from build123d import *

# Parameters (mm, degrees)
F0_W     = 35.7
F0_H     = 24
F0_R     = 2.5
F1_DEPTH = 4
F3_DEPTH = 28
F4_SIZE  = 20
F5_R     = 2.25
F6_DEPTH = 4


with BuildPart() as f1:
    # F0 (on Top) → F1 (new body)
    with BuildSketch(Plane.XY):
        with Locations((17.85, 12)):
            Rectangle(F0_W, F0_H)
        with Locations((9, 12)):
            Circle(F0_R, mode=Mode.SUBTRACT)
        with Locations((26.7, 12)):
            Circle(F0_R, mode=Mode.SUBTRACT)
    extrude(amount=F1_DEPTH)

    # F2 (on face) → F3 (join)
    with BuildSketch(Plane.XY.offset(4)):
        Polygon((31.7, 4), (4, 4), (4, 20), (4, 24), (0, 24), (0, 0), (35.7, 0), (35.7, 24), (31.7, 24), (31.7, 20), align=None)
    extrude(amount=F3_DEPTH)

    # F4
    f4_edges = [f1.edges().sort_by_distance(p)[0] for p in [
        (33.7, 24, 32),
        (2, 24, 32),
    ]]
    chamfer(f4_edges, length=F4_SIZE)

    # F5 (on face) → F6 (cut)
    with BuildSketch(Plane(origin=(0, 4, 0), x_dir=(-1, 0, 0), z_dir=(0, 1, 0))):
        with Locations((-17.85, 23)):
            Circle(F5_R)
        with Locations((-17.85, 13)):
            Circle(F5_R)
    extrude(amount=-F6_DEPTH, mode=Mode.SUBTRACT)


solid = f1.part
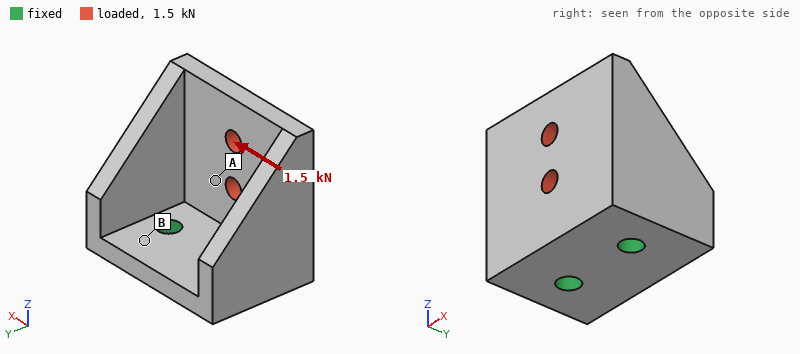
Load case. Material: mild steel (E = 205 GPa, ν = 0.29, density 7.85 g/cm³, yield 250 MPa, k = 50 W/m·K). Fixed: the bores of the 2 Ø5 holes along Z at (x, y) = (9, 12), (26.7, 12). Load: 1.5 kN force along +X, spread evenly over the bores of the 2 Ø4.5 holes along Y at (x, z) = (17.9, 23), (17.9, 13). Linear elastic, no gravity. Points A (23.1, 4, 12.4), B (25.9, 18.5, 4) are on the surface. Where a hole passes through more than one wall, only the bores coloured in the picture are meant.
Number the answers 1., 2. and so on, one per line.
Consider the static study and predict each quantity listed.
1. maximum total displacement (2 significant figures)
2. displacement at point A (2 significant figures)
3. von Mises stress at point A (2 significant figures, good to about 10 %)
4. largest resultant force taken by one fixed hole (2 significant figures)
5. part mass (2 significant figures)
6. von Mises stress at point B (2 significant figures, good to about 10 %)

1. 27 µm
2. 9.4 µm
3. 42 MPa
4. 1.4 kN
5. 79 g
6. 18 MPa
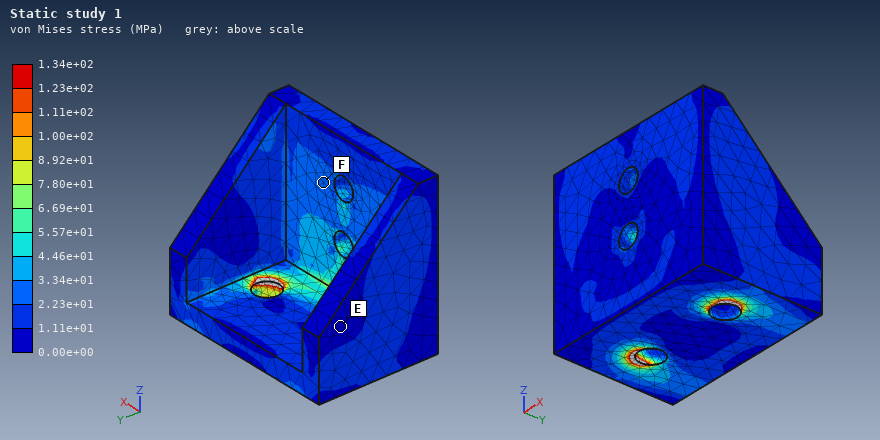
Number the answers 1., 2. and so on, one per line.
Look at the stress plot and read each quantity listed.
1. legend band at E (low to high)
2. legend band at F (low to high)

1. 0.00e+00 to 1.11e+01 MPa
2. 2.23e+01 to 3.34e+01 MPa
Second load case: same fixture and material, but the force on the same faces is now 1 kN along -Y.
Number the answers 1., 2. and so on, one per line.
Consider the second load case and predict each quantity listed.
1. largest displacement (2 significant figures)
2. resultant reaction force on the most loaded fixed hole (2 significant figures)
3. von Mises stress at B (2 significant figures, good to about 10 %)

1. 43 µm
2. 530 N
3. 40 MPa
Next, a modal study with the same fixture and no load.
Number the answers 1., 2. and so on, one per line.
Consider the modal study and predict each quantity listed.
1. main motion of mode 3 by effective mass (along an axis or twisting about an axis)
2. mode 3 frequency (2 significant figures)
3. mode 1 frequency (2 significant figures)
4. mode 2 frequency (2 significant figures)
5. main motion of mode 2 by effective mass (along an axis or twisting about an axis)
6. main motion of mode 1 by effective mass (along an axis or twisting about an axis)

1. along X
2. 12 kHz
3. 4800 Hz
4. 5900 Hz
5. along X
6. along Y
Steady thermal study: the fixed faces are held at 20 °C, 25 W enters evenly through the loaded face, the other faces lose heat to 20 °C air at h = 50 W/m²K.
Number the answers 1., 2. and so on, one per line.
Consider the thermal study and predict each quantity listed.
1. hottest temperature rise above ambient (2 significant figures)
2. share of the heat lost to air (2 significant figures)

1. 60 K
2. 25 %
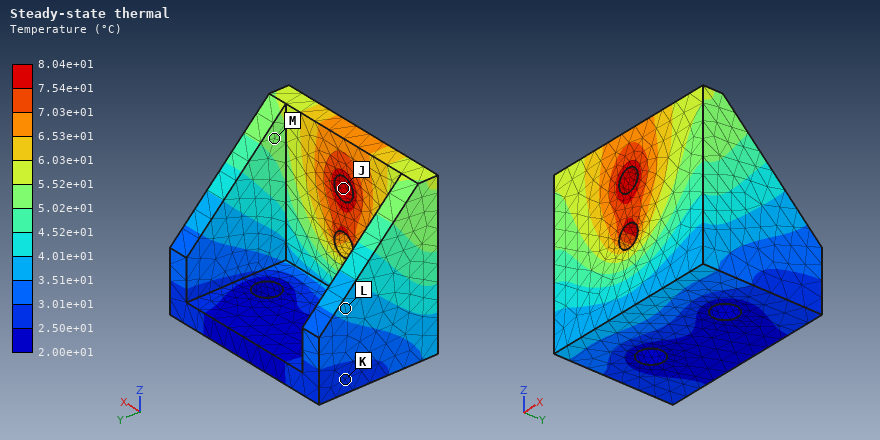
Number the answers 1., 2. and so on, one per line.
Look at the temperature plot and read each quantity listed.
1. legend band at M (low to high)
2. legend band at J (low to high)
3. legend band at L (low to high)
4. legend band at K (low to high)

1. 5.02e+01 to 5.52e+01 °C
2. 7.54e+01 to 8.04e+01 °C
3. 3.51e+01 to 4.01e+01 °C
4. 2.50e+01 to 3.01e+01 °C
